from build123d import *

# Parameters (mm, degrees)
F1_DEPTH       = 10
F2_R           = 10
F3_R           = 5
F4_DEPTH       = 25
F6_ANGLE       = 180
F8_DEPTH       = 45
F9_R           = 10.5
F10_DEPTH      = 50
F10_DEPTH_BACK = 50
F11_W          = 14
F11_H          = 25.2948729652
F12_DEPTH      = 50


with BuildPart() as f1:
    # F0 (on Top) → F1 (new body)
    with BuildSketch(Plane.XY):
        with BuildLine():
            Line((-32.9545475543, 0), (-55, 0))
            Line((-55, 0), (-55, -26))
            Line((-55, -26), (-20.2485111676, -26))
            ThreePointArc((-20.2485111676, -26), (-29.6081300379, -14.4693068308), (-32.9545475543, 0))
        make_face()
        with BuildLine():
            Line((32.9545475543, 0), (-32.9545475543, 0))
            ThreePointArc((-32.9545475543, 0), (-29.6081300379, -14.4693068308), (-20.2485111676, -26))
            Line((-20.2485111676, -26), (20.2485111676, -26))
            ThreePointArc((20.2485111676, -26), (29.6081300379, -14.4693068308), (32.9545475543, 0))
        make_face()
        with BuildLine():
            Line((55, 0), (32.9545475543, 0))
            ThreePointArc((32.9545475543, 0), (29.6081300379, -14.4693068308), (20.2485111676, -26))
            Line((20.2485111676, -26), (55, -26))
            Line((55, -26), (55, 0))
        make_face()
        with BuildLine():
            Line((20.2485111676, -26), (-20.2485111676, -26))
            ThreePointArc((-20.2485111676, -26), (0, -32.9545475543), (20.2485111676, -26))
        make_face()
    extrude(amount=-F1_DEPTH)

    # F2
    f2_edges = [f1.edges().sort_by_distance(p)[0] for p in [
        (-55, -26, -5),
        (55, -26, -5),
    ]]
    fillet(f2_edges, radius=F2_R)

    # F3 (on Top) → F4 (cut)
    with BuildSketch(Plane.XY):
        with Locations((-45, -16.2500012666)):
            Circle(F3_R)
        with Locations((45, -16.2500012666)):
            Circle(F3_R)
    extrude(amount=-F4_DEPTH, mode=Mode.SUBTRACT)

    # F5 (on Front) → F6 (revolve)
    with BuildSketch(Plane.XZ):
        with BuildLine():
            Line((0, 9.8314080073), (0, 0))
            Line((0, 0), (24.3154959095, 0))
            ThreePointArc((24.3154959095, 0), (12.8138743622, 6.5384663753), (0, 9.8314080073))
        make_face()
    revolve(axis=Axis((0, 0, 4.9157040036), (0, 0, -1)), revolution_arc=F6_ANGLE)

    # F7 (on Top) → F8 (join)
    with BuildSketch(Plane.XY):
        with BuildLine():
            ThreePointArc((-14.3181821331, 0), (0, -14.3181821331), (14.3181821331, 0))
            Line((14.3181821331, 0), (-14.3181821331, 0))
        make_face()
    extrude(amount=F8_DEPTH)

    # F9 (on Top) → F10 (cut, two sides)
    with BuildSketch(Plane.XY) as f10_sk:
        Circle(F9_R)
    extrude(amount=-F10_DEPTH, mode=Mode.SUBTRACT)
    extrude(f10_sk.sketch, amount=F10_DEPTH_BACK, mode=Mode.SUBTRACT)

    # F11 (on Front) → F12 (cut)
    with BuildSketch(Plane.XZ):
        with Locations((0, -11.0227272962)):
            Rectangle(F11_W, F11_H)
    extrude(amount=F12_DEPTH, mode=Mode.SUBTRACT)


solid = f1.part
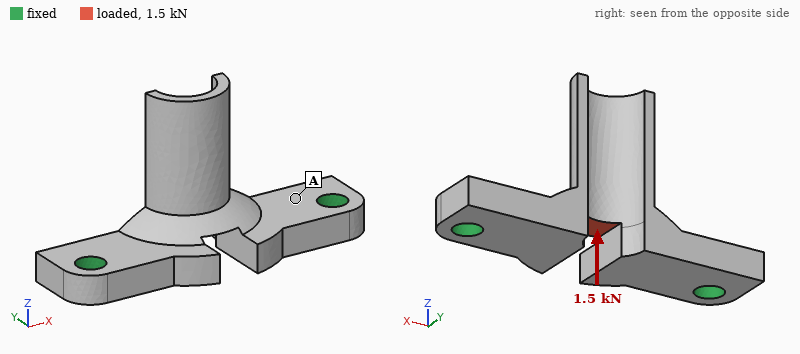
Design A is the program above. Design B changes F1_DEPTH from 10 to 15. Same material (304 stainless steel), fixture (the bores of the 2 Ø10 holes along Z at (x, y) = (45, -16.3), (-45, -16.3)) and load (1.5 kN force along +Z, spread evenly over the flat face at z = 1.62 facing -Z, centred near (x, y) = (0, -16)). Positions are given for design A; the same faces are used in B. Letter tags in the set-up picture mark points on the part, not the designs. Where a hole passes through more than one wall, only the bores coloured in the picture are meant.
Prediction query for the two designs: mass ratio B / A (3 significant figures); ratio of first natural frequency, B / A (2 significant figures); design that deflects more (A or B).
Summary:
1.37
1.2
A
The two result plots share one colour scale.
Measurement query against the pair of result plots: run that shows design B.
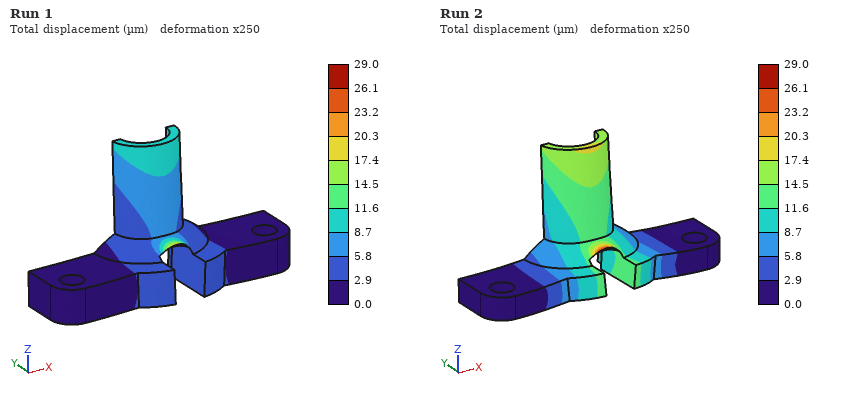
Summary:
Run 1
